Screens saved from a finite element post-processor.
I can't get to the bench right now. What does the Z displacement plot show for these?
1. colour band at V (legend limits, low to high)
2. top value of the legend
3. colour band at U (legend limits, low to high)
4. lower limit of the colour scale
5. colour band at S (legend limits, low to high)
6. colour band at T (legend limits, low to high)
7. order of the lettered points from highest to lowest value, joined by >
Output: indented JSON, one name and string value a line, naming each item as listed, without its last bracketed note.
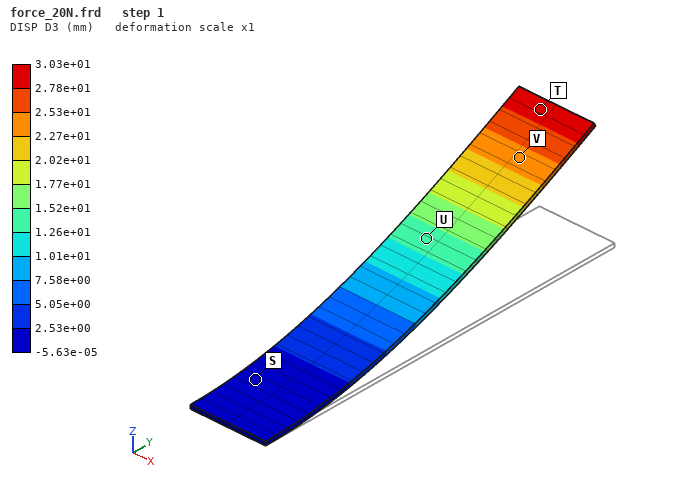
{
  "colour band at V": "2.27e+01 to 2.53e+01 mm",
  "top value of the legend": "3.03e+01 mm",
  "colour band at U": "1.26e+01 to 1.52e+01 mm",
  "lower limit of the colour scale": "-5.63e-05 mm",
  "colour band at S": "-5.63e-05 to 2.53e+00 mm",
  "colour band at T": "2.78e+01 to 3.03e+01 mm",
  "order of the lettered points from highest to lowest value, joined by >": "T > V > U > S"
}
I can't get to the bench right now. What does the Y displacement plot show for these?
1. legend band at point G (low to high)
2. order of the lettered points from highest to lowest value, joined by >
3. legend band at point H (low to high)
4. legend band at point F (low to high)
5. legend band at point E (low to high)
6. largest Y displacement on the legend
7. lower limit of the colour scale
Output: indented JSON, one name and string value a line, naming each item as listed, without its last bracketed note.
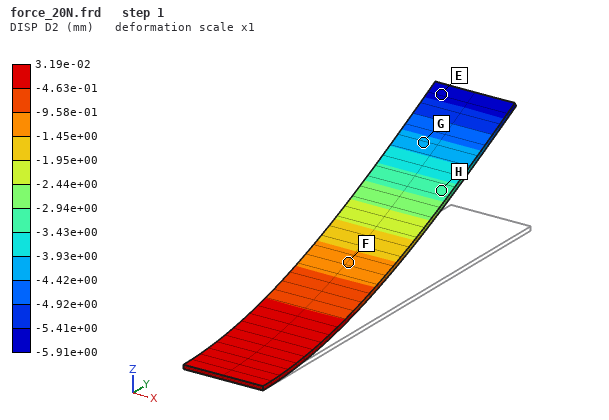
{
  "legend band at point G": "-4.42e+00 to -3.93e+00 mm",
  "order of the lettered points from highest to lowest value, joined by >": "F > H > G > E",
  "legend band at point H": "-3.43e+00 to -2.94e+00 mm",
  "legend band at point F": "-1.45e+00 to -9.58e-01 mm",
  "legend band at point E": "-5.91e+00 to -5.41e+00 mm",
  "largest Y displacement on the legend": "3.19e-02 mm",
  "lower limit of the colour scale": "-5.91e+00 mm"
}
